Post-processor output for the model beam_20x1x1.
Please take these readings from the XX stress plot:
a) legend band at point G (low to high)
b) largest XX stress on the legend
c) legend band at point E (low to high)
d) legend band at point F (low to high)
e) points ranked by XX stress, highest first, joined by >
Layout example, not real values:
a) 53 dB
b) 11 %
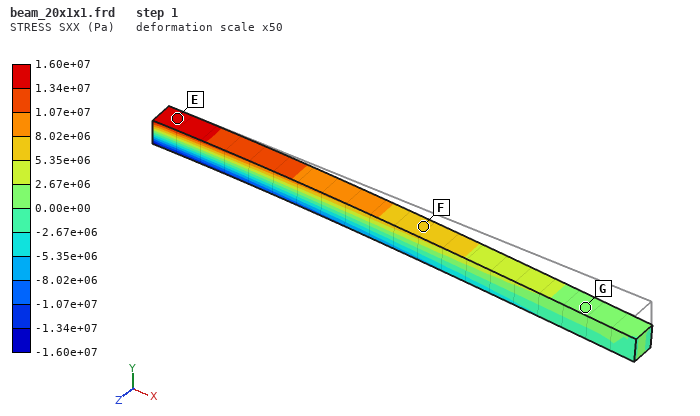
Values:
a) 0.00e+00 to 2.67e+06 Pa
b) 1.60e+07 Pa
c) 1.34e+07 to 1.60e+07 Pa
d) 5.35e+06 to 8.02e+06 Pa
e) E > F > G
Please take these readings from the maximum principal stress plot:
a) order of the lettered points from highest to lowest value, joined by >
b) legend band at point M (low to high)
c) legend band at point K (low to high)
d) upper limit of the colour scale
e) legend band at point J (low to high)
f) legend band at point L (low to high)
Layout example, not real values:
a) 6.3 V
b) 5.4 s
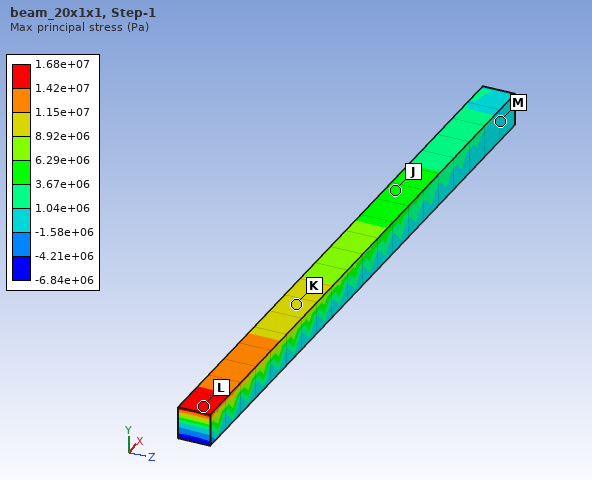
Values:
a) L > K > J > M
b) -1.58e+06 to 1.04e+06 Pa
c) 8.92e+06 to 1.15e+07 Pa
d) 1.68e+07 Pa
e) 3.67e+06 to 6.29e+06 Pa
f) 1.42e+07 to 1.68e+07 Pa
